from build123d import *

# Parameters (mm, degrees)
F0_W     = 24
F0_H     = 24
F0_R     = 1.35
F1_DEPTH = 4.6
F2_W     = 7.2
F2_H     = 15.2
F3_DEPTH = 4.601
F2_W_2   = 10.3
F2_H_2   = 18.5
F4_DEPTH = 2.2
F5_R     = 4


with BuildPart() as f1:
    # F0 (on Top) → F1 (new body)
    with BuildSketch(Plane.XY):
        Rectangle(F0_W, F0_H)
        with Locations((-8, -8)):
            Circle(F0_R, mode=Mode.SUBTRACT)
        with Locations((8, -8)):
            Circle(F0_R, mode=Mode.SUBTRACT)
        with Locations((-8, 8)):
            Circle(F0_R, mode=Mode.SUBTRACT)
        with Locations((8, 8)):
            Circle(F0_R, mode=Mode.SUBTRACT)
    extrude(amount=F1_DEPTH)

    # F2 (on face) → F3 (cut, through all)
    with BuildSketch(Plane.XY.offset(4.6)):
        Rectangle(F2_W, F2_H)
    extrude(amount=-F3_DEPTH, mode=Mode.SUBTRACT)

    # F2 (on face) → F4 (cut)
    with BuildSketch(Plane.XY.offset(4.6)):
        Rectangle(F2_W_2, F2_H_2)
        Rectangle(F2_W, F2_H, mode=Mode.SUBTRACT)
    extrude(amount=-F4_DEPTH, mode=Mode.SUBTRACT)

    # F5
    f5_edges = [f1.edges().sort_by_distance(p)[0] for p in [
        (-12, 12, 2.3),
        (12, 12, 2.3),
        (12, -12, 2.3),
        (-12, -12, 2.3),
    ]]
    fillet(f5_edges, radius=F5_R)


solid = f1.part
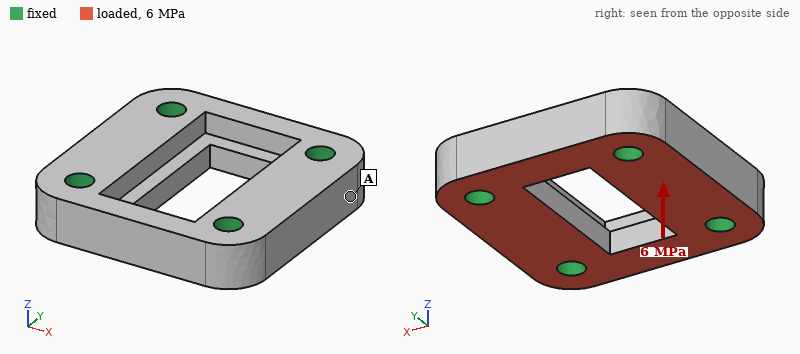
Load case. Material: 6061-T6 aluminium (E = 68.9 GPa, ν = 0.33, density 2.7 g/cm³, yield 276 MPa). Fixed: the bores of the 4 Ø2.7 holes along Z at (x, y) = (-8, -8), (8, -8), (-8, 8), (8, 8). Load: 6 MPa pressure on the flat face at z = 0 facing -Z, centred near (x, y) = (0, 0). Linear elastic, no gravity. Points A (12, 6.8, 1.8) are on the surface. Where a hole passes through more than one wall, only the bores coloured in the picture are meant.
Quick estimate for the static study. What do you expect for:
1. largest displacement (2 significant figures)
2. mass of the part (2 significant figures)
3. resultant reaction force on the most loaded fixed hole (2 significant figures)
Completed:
5.2 µm
4.9 g
650 N
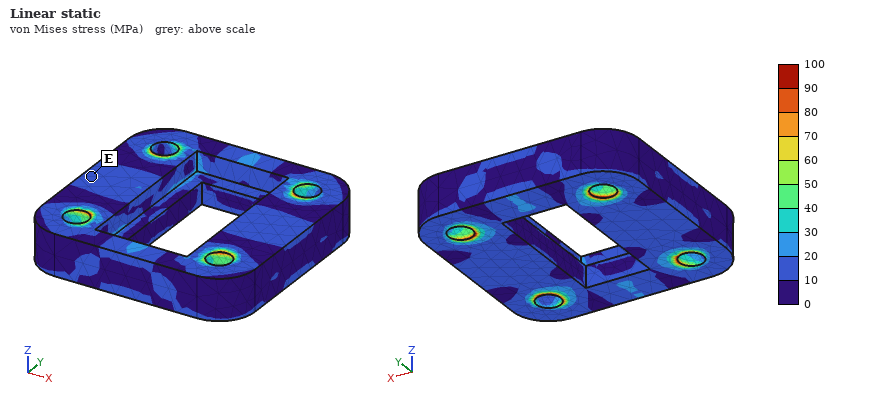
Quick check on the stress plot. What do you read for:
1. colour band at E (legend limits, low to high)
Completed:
10 to 20 MPa
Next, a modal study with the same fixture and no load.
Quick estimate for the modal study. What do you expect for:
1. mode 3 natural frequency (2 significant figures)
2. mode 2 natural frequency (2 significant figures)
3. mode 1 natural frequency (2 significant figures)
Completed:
70 kHz
68 kHz
68 kHz
